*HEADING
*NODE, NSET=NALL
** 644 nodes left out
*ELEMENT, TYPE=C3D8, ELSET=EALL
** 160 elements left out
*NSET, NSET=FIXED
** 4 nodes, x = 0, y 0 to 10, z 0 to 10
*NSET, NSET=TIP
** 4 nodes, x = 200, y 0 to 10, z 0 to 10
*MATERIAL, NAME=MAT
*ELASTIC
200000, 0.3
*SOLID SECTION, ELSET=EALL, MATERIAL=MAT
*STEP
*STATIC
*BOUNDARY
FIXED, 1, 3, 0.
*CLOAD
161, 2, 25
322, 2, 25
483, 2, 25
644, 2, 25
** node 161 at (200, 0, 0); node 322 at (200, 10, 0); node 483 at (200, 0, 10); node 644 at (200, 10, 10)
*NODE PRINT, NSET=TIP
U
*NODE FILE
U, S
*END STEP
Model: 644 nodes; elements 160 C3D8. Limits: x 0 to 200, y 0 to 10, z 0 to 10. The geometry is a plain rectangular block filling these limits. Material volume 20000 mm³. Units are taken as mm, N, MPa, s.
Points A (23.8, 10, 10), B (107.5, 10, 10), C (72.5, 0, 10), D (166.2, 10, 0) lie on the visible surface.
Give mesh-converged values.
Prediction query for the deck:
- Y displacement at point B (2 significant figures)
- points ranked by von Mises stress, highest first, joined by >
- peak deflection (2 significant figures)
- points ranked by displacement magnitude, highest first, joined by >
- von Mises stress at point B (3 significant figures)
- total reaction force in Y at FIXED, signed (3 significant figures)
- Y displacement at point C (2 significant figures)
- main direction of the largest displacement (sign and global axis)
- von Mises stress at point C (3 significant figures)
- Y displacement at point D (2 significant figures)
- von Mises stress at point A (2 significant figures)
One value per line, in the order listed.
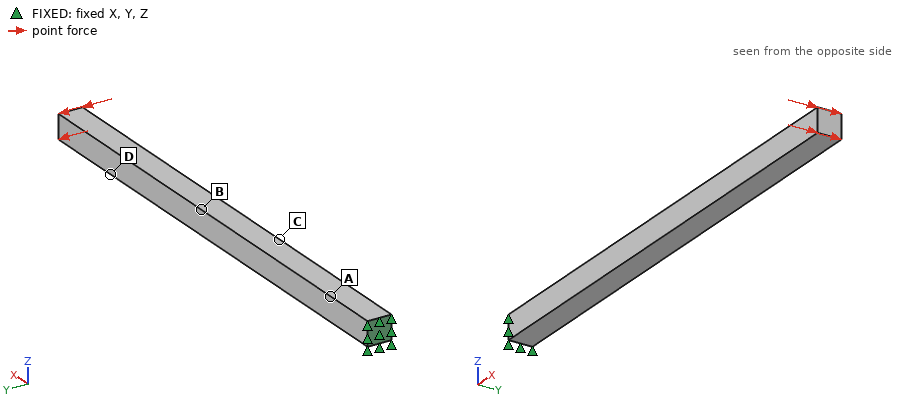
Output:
0.57 mm
A > C > B > D
1.6 mm
D > B > C > A
55.5 MPa
-100 N
0.28 mm
+Y
76.5 MPa
1.2 mm
110 MPa
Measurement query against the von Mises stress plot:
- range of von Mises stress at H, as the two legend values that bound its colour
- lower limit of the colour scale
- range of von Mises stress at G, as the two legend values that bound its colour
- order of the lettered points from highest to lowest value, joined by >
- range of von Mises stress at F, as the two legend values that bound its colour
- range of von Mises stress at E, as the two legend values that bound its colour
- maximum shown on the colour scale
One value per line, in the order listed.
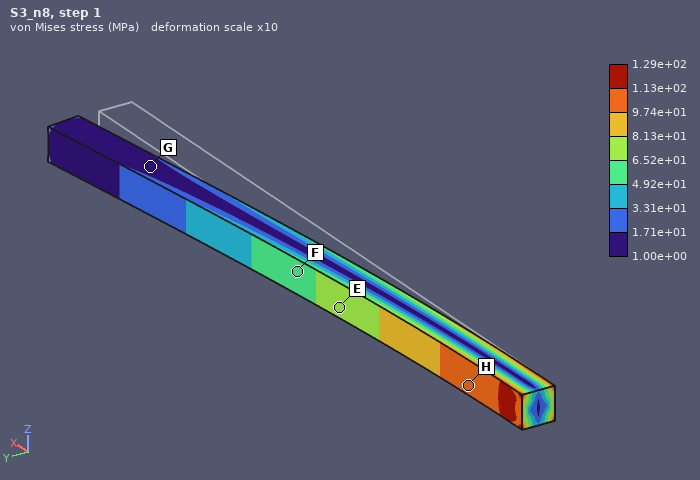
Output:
9.74e+01 to 1.13e+02 MPa
1.00e+00 MPa
1.00e+00 to 1.71e+01 MPa
H > E > F > G
4.92e+01 to 6.52e+01 MPa
6.52e+01 to 8.13e+01 MPa
1.29e+02 MPa
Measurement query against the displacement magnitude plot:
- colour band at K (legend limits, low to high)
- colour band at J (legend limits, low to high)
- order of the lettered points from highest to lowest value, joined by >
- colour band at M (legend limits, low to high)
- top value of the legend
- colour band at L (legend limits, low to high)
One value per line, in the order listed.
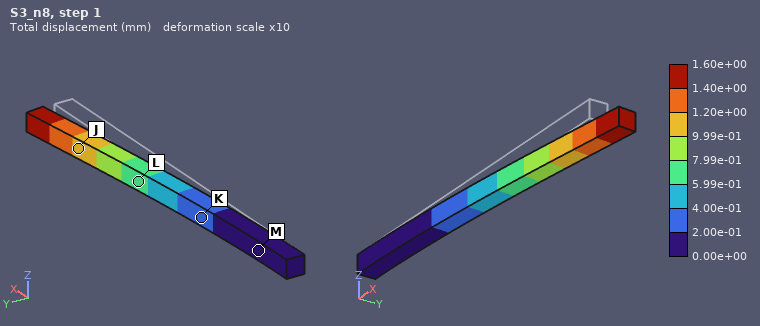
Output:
2.00e-01 to 4.00e-01 mm
9.99e-01 to 1.20e+00 mm
J > L > K > M
0.00e+00 to 2.00e-01 mm
1.60e+00 mm
5.99e-01 to 7.99e-01 mm
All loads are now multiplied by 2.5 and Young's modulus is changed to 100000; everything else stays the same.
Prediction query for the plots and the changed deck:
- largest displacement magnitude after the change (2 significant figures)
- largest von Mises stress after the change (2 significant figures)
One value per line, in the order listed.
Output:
8.0 mm
320 MPa
